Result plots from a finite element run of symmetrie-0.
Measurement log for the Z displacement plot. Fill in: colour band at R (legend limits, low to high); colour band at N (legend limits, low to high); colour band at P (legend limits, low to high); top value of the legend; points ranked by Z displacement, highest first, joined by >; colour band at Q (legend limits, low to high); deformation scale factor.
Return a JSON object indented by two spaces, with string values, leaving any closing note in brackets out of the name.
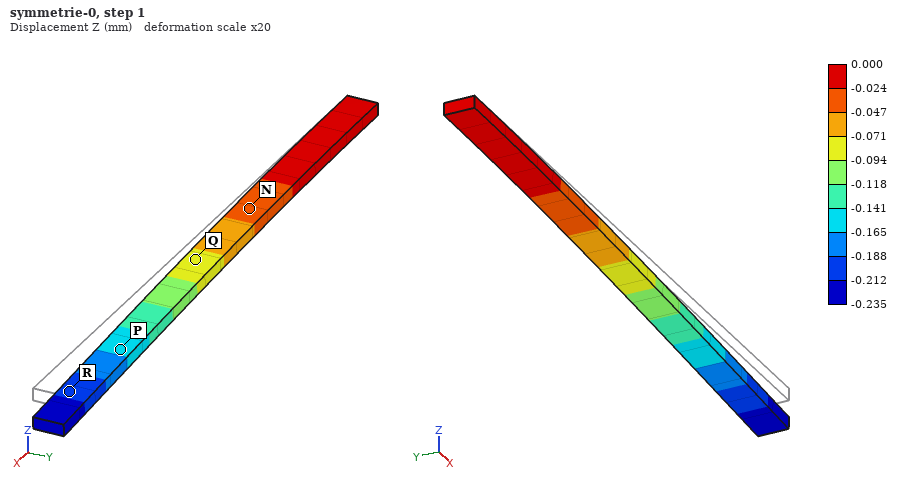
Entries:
{
  "colour band at R": "-0.212 to -0.188 mm",
  "colour band at N": "-0.047 to -0.024 mm",
  "colour band at P": "-0.165 to -0.141 mm",
  "top value of the legend": "0.000 mm",
  "points ranked by Z displacement, highest first, joined by >": "N > Q > P > R",
  "colour band at Q": "-0.094 to -0.071 mm",
  "deformation scale factor": "20"
}
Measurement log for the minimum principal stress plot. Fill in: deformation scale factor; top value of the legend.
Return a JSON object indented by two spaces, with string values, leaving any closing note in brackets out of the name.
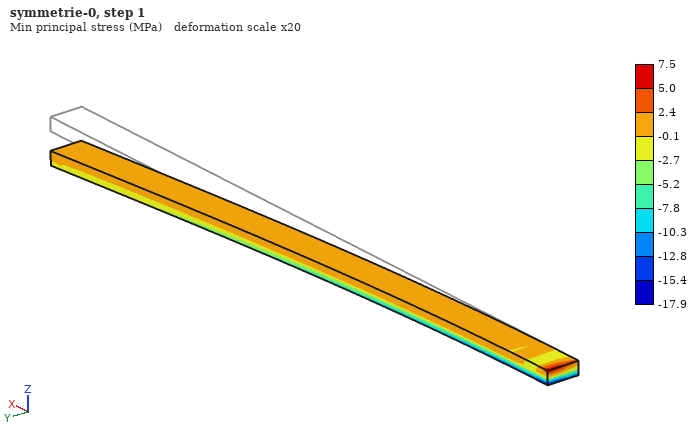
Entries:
{
  "deformation scale factor": "20",
  "top value of the legend": "7.5 MPa"
}
